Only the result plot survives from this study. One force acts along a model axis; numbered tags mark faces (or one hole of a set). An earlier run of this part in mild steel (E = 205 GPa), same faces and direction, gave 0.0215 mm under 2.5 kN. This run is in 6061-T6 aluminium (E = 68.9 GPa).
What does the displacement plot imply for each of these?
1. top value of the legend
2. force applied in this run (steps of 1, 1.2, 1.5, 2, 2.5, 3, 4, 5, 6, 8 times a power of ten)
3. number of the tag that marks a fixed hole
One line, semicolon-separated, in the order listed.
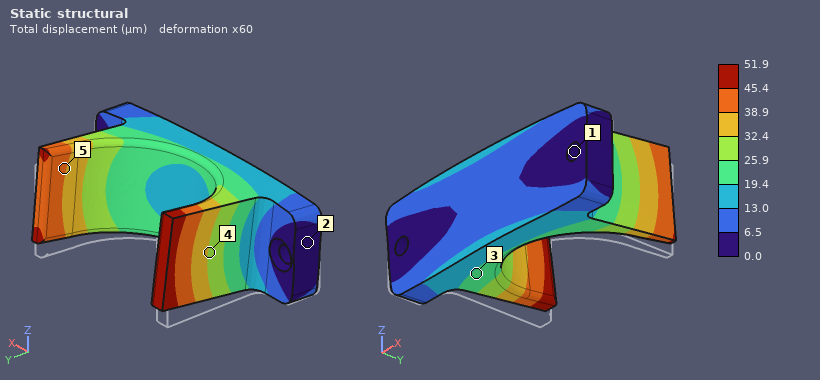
51.9 µm; 2 kN; 1
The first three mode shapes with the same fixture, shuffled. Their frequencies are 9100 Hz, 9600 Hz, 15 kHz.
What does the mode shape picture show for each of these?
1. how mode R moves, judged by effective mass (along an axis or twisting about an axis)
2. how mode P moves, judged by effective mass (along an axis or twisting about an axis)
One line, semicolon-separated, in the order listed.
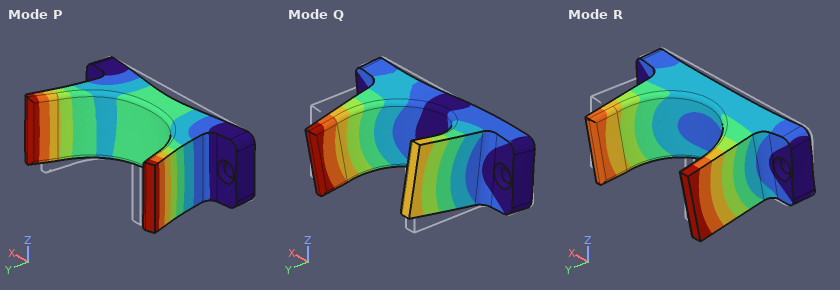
along Z; along Y
